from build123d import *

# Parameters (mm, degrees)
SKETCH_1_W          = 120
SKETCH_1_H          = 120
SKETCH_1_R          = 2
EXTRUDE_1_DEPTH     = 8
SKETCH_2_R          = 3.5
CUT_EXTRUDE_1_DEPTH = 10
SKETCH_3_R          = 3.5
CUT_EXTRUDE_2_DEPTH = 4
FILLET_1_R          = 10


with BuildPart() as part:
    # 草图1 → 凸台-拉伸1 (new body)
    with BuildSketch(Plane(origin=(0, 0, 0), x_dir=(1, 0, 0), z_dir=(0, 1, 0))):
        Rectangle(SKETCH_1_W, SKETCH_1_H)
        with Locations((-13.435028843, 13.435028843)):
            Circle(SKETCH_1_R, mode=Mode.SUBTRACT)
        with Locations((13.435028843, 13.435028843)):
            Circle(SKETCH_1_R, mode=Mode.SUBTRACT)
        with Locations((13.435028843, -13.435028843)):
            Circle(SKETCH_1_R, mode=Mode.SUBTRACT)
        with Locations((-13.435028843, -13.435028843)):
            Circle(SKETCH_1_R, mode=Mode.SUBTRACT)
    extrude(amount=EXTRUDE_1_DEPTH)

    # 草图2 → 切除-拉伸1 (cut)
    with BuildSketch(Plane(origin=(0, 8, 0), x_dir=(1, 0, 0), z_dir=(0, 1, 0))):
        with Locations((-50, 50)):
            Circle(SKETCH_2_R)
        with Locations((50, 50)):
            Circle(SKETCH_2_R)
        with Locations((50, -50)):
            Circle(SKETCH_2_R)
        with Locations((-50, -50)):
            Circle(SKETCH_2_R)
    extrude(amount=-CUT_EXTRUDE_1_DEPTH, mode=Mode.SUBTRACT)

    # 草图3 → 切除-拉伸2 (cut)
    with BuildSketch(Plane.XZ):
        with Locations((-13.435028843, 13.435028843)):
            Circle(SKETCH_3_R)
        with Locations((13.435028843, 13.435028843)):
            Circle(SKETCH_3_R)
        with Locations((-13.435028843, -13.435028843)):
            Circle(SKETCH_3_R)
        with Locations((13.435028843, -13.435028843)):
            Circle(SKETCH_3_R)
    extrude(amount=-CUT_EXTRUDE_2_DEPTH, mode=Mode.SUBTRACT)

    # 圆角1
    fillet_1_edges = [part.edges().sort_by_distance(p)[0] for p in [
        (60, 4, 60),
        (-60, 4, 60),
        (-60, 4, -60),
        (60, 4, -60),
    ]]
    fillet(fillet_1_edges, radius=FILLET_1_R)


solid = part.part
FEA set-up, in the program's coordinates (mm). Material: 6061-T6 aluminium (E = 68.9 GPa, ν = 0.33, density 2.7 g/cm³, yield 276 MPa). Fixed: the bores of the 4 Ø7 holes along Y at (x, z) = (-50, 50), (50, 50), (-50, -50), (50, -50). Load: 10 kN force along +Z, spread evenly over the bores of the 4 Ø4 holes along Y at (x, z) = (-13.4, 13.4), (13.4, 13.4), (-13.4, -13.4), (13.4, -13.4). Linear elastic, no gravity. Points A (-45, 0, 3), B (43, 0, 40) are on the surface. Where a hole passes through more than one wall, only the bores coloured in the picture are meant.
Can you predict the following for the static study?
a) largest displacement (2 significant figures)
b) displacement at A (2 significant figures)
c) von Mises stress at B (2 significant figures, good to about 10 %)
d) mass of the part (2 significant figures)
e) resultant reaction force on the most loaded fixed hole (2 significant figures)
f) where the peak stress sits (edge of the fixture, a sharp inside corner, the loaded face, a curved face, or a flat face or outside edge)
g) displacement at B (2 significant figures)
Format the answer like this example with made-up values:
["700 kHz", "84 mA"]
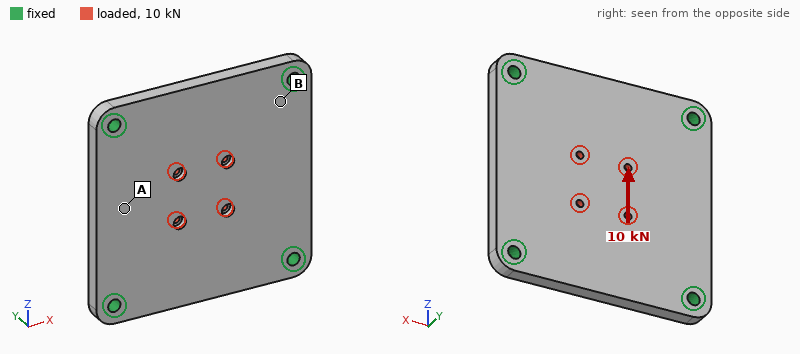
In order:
["17 µm", "4.8 µm", "16 MPa", "300 g", "2.8 kN", "the loaded face", "3.6 µm"]
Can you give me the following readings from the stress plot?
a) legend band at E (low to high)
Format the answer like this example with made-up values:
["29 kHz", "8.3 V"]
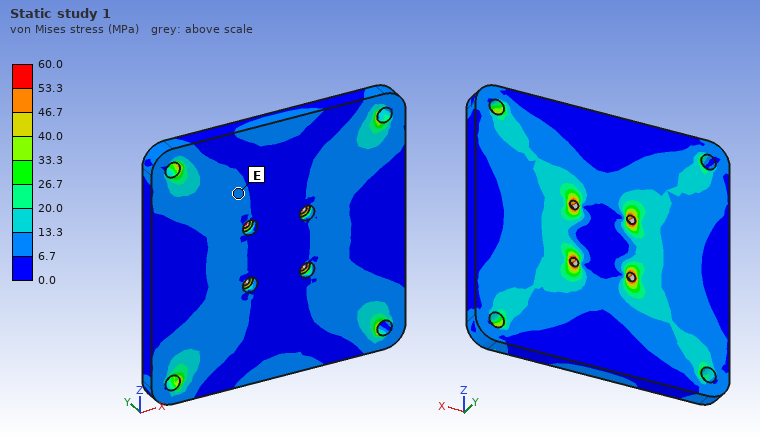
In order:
["6.7 to 13.3 MPa"]
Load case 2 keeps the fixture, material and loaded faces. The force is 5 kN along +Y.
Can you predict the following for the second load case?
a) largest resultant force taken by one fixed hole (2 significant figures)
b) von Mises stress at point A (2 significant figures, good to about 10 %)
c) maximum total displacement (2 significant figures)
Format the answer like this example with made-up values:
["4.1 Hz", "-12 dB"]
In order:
["1.3 kN", "30 MPa", "0.20 mm"]
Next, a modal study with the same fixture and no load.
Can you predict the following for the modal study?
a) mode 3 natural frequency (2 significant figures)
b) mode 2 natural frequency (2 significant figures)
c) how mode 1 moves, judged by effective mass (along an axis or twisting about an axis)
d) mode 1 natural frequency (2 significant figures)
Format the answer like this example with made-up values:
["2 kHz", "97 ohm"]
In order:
["4500 Hz", "4500 Hz", "along Y", "2700 Hz"]
